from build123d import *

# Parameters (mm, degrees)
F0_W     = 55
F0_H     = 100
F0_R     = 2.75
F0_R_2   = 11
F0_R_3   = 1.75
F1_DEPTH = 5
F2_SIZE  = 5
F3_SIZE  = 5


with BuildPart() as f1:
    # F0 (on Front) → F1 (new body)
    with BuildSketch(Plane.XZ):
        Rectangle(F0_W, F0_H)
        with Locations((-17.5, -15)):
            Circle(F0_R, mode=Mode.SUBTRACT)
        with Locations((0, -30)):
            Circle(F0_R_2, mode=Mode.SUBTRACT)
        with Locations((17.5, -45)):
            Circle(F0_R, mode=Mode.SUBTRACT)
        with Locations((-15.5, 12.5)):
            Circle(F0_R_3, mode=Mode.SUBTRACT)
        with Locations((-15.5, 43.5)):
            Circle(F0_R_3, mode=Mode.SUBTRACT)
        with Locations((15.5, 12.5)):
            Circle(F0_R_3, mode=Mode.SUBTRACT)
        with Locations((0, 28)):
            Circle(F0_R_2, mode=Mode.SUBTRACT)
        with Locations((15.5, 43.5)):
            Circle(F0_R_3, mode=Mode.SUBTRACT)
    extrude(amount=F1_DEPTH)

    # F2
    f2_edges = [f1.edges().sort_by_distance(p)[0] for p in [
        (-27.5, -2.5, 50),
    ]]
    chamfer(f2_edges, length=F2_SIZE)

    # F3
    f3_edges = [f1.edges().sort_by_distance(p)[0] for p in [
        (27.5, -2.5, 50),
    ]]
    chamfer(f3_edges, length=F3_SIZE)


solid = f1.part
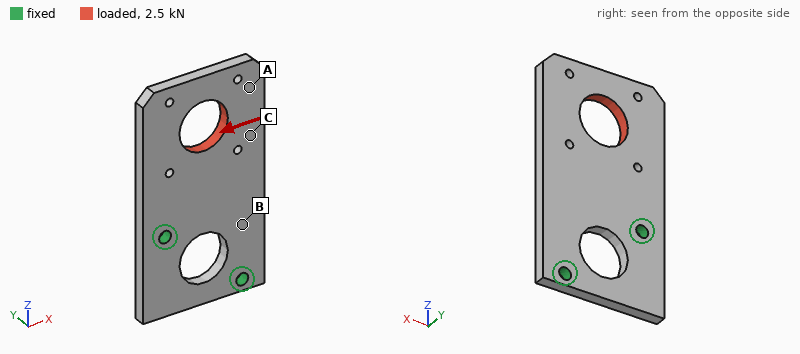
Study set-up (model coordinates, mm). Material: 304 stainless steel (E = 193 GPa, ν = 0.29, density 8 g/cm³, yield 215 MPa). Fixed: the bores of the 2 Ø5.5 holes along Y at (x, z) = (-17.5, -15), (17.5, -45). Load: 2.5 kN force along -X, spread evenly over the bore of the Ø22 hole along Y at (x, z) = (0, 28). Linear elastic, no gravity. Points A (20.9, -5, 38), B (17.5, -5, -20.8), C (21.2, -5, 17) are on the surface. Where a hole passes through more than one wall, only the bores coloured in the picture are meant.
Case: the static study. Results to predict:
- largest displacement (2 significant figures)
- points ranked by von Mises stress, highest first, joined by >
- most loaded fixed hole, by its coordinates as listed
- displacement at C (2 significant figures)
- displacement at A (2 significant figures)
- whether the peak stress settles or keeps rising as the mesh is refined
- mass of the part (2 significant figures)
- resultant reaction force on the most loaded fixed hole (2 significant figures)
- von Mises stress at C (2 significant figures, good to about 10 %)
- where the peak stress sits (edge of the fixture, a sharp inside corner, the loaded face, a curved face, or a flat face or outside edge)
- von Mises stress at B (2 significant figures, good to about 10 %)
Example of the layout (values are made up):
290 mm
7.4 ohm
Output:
33 µm
B > C > A
(-17.5, -15)
17 µm
28 µm
keeps rising
190 g
3.7 kN
17 MPa
edge of the fixture
29 MPa
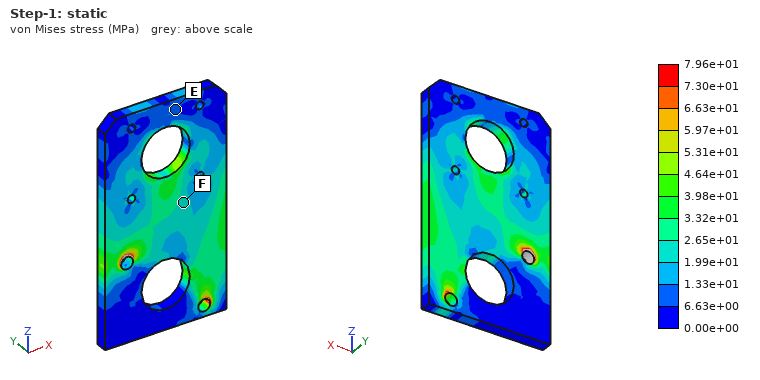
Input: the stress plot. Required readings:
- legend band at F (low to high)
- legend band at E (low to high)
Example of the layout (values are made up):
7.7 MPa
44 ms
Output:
1.99e+01 to 2.65e+01 MPa
6.63e+00 to 1.33e+01 MPa
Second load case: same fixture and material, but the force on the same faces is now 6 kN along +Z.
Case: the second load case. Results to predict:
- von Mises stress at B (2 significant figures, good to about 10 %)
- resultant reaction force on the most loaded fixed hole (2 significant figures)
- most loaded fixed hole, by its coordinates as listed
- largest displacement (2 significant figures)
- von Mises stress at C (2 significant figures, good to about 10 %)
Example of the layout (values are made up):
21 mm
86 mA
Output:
31 MPa
3.3 kN
(-17.5, -15)
16 µm
26 MPa
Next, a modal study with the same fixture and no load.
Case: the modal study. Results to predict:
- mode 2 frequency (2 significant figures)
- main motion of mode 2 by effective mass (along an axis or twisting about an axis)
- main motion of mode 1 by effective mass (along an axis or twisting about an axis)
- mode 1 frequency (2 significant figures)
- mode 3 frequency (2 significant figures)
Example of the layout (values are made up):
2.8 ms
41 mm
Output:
1900 Hz
twisting about Z
along Y
800 Hz
3800 Hz
